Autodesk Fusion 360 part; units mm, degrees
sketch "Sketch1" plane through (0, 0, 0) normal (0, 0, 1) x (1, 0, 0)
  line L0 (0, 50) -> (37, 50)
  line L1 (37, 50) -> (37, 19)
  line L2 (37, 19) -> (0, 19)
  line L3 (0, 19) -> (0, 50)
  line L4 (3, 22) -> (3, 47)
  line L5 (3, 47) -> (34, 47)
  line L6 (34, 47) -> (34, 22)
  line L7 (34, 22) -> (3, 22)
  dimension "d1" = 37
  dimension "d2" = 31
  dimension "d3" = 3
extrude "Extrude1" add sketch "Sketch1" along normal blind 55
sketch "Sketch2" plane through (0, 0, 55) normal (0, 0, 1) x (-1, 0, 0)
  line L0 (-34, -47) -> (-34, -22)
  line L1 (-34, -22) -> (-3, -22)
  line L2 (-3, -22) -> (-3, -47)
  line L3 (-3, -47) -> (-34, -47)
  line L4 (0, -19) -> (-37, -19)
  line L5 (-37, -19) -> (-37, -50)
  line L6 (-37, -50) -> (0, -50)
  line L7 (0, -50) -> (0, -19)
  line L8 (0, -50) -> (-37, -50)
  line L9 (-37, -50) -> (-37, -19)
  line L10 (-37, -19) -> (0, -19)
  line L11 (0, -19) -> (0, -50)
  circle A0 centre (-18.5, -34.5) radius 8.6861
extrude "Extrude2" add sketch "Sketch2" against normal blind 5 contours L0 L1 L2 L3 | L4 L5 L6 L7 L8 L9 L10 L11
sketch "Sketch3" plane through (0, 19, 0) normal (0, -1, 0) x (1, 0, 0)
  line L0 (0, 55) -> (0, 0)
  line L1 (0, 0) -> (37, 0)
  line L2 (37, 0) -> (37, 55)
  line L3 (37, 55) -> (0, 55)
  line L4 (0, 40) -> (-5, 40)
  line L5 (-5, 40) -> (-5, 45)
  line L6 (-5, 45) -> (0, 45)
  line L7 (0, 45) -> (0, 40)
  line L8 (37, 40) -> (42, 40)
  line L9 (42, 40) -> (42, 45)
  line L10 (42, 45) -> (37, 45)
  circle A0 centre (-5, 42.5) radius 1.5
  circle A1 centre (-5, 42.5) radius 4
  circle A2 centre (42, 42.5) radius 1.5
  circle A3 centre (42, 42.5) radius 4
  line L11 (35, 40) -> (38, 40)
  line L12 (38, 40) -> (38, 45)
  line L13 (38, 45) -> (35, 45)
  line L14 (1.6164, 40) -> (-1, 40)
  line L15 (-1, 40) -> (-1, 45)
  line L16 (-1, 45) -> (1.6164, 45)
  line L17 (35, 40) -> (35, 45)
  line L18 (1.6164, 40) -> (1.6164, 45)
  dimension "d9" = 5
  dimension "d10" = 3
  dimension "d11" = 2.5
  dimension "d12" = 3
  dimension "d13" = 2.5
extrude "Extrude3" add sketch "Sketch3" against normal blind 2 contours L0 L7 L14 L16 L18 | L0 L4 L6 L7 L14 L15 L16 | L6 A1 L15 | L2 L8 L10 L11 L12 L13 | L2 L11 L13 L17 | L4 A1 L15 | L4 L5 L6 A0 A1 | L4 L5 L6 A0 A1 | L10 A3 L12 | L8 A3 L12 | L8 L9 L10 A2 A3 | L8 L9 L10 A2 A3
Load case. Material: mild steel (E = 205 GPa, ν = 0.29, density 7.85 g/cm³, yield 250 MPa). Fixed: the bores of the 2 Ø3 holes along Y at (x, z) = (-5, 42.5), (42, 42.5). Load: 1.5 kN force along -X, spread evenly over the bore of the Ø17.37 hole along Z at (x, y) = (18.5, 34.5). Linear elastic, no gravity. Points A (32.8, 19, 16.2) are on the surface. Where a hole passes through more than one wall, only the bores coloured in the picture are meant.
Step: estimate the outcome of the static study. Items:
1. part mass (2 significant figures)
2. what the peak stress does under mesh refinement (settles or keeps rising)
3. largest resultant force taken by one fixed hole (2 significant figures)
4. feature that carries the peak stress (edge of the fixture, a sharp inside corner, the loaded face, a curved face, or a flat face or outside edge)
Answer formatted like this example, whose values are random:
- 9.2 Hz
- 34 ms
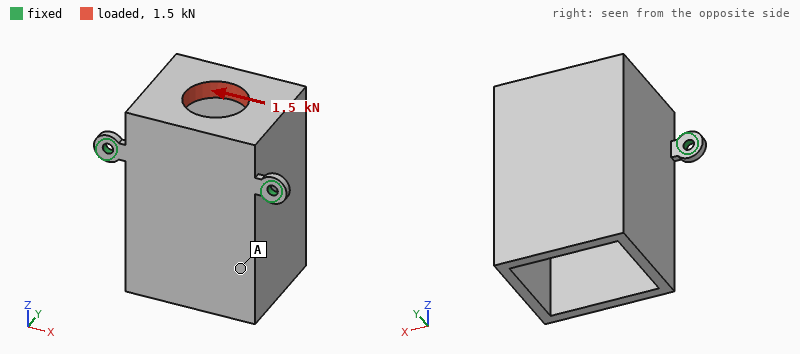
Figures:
- 180 g
- keeps rising
- 990 N
- edge of the fixture
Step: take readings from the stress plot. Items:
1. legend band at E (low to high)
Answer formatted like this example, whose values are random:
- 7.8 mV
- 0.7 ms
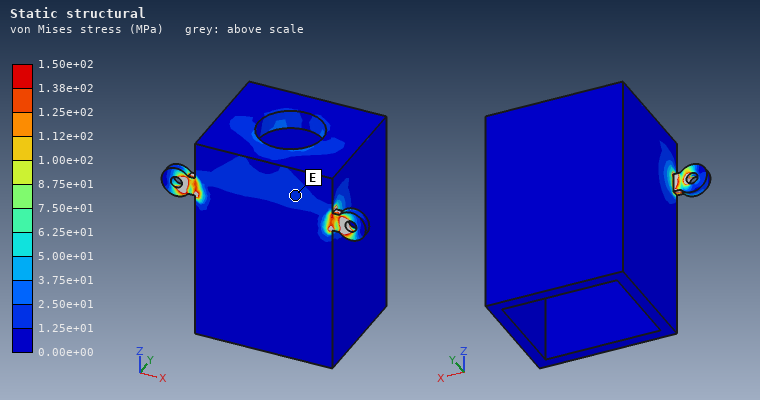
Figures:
- 1.25e+01 to 2.50e+01 MPa
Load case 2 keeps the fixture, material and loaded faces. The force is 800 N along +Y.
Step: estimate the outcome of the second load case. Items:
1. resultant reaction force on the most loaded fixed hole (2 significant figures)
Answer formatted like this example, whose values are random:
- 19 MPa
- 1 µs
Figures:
- 430 N
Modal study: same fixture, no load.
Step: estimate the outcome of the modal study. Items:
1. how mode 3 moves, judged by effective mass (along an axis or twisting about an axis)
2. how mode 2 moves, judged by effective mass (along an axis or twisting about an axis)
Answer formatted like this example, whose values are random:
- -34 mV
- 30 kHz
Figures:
- along Y
- along X
